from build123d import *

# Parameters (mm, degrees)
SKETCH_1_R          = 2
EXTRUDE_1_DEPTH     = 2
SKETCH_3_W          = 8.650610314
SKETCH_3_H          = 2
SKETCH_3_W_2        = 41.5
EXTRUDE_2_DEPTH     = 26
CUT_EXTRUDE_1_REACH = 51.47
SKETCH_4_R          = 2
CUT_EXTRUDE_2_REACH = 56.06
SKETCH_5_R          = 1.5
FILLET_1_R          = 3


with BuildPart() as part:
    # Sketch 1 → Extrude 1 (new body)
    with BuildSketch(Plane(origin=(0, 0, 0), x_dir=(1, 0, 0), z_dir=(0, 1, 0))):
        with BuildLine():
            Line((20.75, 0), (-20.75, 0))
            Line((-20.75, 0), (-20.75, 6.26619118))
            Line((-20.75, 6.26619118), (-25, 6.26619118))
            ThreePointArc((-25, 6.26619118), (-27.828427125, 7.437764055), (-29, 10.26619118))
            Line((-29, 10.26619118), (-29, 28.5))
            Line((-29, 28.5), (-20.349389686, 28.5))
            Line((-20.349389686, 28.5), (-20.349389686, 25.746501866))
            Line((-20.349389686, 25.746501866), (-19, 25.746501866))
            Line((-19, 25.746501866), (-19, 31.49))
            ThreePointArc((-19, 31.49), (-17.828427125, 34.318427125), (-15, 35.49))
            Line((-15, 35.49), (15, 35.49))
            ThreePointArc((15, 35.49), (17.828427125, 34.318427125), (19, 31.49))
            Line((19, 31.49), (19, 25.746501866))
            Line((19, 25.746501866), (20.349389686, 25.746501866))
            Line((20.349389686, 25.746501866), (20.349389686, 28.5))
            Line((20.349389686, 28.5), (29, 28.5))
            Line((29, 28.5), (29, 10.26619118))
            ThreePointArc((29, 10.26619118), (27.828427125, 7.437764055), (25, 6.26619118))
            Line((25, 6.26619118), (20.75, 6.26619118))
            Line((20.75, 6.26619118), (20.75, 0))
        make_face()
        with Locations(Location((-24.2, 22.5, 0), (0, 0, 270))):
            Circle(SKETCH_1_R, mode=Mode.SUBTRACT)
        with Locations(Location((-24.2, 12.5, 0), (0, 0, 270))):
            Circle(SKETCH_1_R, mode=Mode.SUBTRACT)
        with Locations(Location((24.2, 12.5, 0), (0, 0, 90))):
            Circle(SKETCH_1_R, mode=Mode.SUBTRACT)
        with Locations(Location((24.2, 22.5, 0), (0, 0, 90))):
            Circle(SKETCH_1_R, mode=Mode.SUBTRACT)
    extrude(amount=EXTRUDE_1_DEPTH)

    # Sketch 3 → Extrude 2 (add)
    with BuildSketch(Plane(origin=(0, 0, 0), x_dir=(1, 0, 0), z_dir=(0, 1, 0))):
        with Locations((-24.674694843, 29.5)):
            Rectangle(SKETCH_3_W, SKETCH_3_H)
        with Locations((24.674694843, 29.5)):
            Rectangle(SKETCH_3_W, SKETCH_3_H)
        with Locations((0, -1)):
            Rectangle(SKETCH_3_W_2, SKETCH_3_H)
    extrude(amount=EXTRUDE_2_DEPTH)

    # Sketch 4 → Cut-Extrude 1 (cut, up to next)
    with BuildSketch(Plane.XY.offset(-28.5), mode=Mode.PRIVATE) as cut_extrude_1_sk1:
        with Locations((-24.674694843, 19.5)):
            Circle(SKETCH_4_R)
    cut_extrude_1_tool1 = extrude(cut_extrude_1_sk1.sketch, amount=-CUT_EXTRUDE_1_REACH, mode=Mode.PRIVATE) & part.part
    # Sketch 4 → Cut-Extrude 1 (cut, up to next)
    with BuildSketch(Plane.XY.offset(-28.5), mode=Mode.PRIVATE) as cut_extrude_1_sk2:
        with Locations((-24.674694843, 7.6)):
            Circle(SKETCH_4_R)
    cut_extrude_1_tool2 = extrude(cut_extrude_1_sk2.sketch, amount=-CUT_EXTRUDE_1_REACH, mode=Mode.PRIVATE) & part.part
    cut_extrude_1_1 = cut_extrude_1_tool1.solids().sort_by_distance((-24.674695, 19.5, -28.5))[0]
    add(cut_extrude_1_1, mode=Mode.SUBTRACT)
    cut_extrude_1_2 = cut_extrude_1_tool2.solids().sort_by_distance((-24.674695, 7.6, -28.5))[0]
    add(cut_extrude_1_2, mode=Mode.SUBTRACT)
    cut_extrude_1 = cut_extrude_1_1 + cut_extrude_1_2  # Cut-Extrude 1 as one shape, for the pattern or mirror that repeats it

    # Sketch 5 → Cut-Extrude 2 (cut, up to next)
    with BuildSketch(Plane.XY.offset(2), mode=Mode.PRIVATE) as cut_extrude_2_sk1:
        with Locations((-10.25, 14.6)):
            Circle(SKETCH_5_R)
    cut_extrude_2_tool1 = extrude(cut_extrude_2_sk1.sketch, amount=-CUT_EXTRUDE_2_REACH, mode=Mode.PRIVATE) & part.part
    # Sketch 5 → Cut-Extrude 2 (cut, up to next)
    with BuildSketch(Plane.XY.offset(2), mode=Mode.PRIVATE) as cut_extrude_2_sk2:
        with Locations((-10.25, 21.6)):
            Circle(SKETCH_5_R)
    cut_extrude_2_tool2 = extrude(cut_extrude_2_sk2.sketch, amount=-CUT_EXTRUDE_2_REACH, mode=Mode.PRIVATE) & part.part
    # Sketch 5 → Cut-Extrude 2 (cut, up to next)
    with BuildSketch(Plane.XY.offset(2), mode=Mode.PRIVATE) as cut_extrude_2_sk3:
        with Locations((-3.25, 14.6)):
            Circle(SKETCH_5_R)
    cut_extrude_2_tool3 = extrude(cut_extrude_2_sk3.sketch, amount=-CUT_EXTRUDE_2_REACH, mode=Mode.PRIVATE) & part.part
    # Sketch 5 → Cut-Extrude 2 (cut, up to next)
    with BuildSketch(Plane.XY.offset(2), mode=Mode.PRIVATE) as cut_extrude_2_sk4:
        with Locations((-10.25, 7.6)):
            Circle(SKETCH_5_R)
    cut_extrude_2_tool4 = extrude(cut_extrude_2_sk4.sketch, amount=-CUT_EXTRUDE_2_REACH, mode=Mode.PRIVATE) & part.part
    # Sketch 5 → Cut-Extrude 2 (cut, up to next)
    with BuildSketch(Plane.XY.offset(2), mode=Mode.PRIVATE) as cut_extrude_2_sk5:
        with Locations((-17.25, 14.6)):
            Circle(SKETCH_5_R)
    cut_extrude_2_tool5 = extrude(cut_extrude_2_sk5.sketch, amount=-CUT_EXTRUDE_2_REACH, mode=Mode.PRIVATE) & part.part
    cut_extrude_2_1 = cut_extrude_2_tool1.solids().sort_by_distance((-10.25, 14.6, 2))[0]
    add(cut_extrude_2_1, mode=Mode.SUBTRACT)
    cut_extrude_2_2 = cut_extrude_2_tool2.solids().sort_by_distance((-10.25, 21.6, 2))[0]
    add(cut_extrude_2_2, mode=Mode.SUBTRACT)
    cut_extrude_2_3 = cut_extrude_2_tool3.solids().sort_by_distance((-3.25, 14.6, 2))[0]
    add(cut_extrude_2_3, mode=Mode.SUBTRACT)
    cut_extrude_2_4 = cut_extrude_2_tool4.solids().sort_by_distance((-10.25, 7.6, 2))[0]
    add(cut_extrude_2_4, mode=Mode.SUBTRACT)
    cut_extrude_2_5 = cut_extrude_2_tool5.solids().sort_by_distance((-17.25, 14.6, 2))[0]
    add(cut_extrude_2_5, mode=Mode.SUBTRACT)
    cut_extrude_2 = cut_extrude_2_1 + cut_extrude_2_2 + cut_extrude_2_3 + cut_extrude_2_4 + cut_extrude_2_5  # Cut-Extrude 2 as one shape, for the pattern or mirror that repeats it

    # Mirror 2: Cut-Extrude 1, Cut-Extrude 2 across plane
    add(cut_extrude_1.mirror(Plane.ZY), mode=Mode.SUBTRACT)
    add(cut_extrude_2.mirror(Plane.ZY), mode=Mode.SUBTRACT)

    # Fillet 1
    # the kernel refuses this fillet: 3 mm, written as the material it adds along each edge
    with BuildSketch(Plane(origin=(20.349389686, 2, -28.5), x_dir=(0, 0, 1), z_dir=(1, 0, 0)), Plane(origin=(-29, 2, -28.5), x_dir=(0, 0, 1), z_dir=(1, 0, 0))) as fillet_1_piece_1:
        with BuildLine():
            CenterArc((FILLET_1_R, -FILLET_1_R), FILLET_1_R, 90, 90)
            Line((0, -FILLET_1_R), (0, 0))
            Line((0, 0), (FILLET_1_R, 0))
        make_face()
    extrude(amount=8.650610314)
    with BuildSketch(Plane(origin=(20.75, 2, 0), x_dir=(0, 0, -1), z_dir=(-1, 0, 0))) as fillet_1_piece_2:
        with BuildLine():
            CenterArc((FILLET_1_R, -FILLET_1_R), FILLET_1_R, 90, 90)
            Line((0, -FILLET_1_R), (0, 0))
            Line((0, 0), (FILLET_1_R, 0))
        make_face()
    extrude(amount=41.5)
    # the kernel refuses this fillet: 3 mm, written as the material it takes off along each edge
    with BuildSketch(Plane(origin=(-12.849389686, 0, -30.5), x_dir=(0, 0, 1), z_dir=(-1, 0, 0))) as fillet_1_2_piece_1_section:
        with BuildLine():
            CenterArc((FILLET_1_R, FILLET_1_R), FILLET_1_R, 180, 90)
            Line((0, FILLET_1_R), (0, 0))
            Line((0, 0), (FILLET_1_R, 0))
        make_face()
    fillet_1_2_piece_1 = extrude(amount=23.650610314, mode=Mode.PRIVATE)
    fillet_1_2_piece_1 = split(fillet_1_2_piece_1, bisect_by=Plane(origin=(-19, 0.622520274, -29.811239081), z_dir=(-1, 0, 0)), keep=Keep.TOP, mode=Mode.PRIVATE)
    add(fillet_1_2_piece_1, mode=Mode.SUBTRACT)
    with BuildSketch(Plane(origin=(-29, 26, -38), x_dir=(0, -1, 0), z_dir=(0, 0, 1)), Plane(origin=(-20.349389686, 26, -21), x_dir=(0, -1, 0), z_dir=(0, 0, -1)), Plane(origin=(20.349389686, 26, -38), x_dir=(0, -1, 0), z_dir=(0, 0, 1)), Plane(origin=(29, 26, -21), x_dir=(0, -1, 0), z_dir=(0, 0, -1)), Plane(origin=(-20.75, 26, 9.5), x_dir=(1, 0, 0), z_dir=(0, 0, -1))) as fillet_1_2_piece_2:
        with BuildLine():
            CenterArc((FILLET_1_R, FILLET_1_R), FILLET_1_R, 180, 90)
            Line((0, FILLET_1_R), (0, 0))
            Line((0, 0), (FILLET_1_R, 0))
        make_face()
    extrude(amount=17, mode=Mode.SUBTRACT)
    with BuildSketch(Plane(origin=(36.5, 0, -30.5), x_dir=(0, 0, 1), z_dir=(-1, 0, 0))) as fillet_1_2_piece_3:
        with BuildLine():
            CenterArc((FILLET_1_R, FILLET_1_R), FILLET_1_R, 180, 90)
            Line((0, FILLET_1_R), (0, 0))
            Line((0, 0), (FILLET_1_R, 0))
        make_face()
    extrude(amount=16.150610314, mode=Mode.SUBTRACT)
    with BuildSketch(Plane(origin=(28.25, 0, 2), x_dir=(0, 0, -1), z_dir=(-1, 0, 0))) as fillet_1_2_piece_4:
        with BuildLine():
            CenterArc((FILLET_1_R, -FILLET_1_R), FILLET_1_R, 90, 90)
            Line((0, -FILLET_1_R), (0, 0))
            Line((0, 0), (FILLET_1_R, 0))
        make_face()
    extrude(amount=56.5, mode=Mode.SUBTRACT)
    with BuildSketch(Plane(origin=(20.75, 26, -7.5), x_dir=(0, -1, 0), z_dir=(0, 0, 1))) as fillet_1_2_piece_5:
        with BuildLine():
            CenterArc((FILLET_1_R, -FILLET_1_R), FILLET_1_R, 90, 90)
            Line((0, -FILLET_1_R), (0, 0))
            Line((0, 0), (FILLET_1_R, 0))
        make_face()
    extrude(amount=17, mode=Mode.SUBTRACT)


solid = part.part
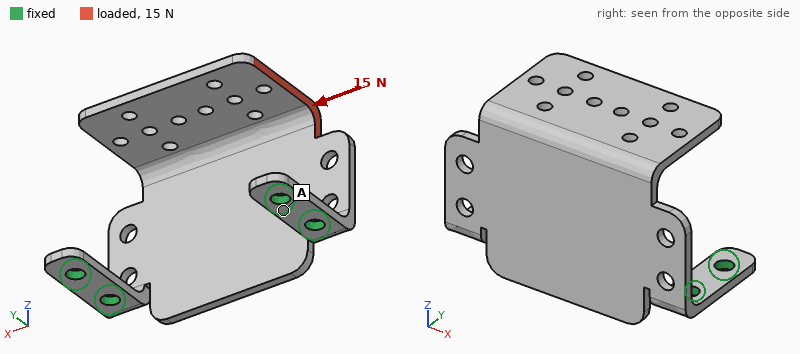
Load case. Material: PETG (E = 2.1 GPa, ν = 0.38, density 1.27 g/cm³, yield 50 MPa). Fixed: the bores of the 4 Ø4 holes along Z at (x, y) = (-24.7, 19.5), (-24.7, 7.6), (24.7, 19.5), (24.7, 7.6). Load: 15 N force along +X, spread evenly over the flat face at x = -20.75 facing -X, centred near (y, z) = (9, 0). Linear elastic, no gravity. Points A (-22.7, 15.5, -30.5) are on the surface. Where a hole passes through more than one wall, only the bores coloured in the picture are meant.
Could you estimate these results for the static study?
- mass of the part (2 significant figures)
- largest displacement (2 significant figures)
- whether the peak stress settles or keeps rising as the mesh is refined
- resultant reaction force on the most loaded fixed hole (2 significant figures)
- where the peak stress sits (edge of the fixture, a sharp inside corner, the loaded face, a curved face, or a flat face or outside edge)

8.0 g
0.78 mm
keeps rising
12 N
edge of the fixture
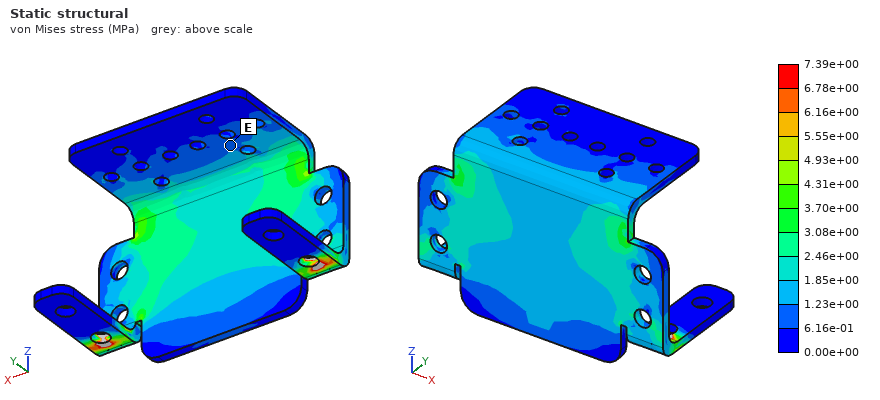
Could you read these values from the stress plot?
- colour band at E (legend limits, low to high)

6.16e-01 to 1.23e+00 MPa
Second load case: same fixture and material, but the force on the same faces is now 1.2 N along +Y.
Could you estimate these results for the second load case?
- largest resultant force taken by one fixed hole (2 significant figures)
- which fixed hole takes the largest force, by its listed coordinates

1.1 N
(-24.7, 7.6)
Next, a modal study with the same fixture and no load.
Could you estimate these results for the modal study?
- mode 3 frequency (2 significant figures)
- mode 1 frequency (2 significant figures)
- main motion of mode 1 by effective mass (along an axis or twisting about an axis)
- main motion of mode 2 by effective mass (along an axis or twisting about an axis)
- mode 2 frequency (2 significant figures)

480 Hz
120 Hz
along Y
along X
370 Hz
